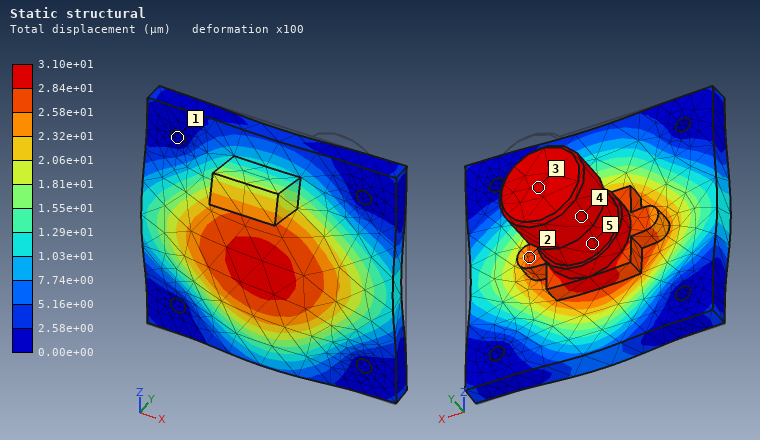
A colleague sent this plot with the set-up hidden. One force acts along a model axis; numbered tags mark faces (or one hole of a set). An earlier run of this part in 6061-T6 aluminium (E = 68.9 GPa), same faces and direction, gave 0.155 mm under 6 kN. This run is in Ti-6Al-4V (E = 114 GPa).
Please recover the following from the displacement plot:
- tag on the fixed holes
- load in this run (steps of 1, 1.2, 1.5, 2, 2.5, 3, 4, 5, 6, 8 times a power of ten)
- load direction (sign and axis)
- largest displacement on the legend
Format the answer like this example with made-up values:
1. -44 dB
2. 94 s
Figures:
1. 1
2. 2 kN
3. -Y
4. 3.10e+01 µm
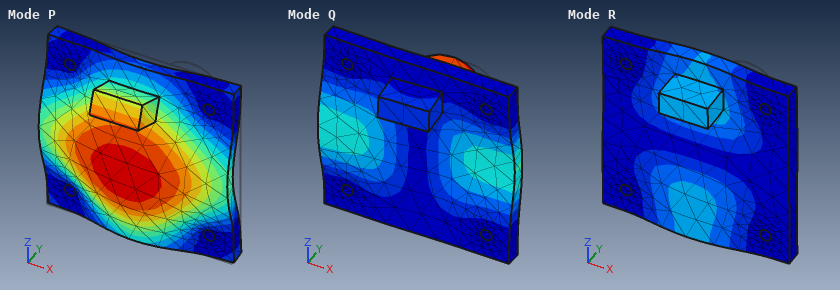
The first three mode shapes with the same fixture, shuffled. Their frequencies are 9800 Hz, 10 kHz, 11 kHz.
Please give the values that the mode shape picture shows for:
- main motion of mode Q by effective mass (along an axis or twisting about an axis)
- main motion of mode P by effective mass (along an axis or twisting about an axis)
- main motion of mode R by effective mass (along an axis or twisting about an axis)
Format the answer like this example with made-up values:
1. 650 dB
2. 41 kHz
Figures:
1. along X
2. along Y
3. along Z
